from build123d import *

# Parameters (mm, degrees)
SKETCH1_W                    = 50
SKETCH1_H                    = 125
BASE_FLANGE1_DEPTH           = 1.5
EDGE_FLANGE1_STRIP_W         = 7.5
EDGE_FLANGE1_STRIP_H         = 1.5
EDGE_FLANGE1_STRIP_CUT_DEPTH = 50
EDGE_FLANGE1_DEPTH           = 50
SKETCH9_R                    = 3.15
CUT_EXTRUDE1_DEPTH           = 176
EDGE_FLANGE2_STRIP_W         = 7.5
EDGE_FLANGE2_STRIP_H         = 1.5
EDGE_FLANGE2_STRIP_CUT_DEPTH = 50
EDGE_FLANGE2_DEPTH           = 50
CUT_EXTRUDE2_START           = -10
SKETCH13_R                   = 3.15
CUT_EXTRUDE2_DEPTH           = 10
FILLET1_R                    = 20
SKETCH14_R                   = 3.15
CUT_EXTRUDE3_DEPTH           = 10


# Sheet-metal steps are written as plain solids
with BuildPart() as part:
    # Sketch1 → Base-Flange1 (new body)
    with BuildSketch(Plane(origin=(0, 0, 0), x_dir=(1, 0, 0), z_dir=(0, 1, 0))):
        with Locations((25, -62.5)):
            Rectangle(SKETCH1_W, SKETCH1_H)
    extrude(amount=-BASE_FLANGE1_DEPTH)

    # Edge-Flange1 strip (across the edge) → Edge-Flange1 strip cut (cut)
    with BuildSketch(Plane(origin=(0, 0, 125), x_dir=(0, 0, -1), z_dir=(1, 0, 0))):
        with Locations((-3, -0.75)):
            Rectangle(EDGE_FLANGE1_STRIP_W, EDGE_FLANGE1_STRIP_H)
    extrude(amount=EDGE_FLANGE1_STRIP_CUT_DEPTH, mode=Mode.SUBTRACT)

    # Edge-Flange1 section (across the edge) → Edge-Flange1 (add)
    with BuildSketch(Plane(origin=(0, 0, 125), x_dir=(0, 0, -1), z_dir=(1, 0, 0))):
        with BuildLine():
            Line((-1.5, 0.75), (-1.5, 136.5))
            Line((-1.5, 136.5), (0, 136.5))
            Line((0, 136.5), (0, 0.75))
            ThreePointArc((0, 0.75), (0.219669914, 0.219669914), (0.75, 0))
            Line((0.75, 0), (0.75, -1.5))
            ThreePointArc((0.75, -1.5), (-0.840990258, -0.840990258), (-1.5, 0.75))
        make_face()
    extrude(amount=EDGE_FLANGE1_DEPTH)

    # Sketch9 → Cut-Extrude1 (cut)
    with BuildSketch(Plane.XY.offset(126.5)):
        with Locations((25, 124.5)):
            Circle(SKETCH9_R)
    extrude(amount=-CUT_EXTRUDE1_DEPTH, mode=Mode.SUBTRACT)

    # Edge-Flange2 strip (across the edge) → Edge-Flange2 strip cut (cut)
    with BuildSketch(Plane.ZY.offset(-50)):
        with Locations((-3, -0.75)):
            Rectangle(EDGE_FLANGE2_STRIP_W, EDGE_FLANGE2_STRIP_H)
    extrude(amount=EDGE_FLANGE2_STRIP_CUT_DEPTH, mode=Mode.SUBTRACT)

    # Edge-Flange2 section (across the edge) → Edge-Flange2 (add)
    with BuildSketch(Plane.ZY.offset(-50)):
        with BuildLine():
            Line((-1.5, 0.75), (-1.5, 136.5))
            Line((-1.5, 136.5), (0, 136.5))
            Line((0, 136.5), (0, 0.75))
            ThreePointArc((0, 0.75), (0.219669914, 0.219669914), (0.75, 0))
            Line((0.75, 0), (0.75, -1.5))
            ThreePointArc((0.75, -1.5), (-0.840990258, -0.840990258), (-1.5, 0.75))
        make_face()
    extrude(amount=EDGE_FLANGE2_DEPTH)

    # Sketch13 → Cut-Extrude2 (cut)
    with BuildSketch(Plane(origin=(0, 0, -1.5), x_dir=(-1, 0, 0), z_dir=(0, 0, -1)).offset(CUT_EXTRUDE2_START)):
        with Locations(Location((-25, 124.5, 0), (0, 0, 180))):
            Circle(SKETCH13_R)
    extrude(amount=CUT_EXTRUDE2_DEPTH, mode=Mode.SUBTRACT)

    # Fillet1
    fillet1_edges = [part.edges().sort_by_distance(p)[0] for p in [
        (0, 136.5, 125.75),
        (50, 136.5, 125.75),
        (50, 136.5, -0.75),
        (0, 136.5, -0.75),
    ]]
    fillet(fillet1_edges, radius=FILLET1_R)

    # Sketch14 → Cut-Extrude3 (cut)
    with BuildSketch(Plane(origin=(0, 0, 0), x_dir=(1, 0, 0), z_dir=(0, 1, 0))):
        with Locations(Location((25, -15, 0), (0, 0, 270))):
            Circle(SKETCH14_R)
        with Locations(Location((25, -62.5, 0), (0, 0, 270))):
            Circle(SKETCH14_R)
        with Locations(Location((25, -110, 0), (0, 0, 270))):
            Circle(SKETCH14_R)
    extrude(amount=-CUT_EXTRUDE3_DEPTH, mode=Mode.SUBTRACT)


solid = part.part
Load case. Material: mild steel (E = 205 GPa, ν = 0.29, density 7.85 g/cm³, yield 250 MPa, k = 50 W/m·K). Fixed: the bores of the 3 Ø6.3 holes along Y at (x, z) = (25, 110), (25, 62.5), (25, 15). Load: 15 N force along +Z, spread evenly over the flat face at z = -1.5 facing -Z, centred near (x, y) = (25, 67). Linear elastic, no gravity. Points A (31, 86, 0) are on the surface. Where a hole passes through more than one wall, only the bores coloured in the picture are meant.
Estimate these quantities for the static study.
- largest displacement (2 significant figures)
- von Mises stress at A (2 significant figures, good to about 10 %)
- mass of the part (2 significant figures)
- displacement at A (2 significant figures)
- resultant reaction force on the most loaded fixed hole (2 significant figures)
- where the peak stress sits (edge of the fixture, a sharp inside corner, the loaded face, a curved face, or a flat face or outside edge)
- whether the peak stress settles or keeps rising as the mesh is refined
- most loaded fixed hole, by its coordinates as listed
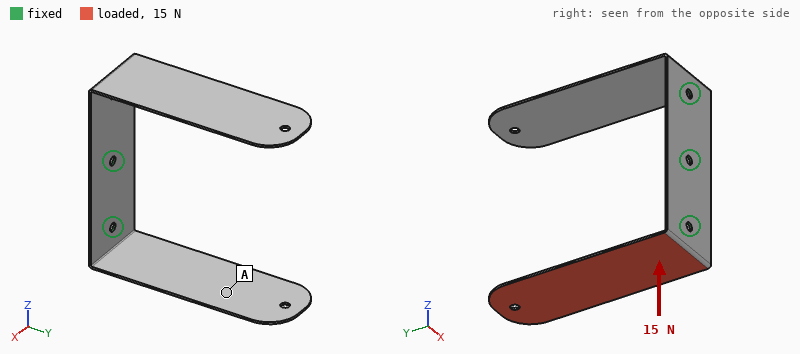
2.3 mm
7.0 MPa
230 g
1.3 mm
14 N
edge of the fixture
keeps rising
(25, 15)
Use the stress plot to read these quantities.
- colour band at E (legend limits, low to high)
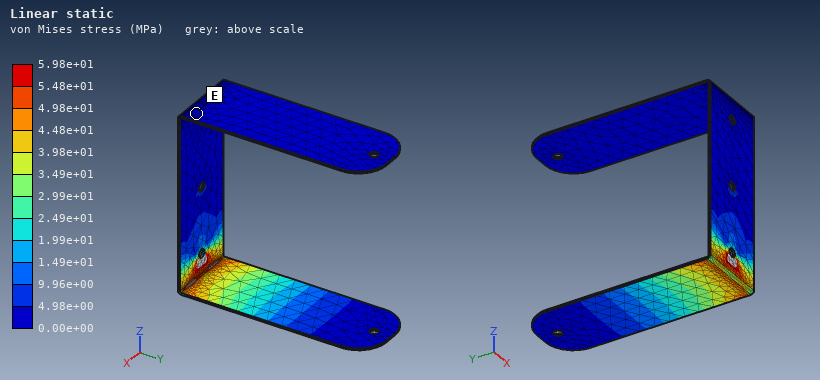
0.00e+00 to 4.98e+00 MPa
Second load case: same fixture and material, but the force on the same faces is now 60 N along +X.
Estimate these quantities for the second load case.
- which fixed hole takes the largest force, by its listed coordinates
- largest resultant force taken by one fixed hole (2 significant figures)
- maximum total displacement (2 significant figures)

(25, 15)
73 N
1.5 mm
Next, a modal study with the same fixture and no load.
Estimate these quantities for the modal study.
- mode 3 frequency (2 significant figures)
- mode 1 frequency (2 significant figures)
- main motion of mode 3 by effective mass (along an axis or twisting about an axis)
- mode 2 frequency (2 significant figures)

140 Hz
58 Hz
along X
58 Hz
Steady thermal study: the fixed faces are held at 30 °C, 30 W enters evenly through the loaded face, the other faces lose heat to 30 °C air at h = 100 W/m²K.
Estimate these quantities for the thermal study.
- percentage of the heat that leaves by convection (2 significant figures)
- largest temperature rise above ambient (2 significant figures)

94 %
42 K
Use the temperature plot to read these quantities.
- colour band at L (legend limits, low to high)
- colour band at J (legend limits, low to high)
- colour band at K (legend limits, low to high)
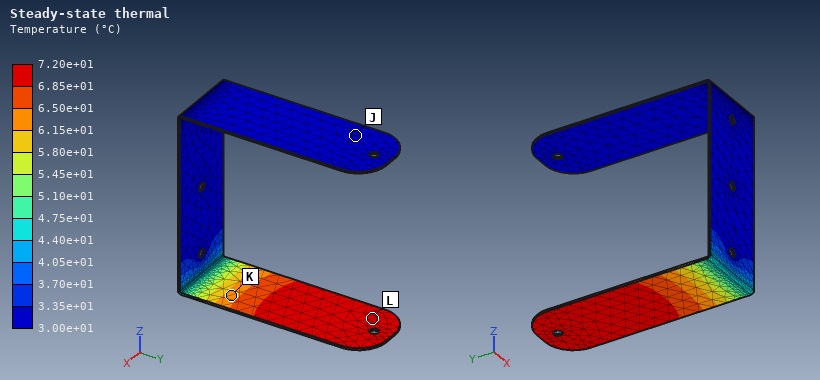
6.85e+01 to 7.20e+01 °C
3.00e+01 to 3.35e+01 °C
6.15e+01 to 6.50e+01 °C
